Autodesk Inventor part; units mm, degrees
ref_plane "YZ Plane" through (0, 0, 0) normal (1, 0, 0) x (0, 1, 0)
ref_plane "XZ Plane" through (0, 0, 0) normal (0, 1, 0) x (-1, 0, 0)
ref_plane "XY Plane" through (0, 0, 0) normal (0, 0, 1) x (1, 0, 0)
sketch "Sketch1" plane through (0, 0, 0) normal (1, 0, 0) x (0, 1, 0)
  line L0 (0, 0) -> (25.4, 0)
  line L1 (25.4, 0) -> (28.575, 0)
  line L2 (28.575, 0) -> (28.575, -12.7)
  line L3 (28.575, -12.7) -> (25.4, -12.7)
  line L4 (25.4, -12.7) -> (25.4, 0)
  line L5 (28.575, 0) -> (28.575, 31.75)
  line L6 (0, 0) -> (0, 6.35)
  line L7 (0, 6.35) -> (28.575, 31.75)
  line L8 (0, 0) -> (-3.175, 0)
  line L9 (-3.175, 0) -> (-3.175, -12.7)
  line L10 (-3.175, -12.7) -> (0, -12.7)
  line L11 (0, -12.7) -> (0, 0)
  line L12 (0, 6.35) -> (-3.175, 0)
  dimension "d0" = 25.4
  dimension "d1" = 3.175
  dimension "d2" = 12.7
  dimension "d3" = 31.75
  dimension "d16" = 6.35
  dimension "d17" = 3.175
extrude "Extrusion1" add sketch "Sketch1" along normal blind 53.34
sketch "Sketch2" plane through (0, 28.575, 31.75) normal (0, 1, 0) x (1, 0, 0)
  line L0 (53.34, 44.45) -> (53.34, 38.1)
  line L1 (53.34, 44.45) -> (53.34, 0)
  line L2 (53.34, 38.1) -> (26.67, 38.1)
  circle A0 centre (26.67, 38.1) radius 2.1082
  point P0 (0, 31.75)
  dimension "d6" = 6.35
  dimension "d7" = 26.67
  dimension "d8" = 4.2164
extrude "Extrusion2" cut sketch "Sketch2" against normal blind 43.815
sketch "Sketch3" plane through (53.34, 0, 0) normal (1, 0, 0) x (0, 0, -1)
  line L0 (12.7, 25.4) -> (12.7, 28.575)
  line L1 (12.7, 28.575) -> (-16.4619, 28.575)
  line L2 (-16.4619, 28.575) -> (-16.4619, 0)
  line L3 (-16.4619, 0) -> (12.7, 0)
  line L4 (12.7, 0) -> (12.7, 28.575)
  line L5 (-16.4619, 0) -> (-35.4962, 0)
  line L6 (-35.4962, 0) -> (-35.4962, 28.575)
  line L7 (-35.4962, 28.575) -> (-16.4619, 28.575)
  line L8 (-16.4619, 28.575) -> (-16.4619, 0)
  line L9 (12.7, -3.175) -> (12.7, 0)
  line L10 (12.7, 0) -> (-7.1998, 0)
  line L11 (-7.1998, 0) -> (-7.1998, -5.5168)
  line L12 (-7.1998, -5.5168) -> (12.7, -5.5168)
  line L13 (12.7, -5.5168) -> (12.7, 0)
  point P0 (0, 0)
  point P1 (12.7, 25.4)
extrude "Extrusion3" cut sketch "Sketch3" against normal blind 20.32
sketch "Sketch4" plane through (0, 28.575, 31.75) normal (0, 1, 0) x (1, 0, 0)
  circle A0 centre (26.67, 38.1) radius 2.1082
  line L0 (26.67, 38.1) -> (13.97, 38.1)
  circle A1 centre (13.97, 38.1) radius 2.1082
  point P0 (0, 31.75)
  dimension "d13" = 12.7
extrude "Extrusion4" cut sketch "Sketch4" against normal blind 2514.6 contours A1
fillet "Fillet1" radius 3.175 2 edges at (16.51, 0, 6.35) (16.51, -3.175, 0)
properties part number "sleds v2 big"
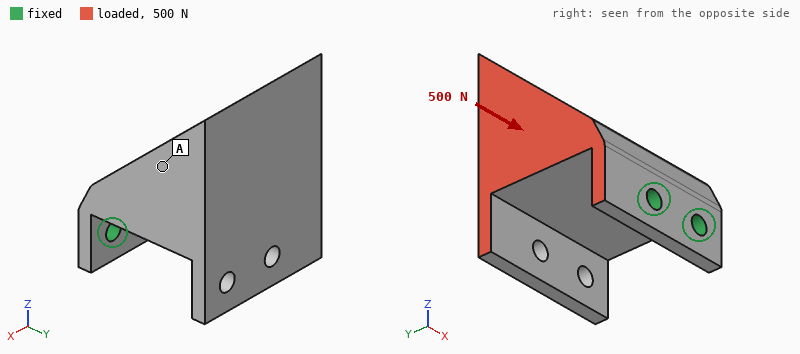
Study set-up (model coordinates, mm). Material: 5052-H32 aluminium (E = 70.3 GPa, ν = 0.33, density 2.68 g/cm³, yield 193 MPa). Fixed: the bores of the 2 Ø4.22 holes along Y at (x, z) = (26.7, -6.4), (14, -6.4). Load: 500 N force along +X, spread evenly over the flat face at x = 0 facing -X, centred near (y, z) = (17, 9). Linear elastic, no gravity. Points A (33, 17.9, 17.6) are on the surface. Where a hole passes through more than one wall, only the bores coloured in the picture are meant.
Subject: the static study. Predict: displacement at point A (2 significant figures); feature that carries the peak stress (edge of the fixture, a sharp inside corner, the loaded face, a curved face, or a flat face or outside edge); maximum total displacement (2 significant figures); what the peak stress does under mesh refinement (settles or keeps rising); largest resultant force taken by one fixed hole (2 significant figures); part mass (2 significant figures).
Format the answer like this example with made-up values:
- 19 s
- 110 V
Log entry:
- 40 µm
- edge of the fixture
- 71 µm
- keeps rising
- 750 N
- 56 g
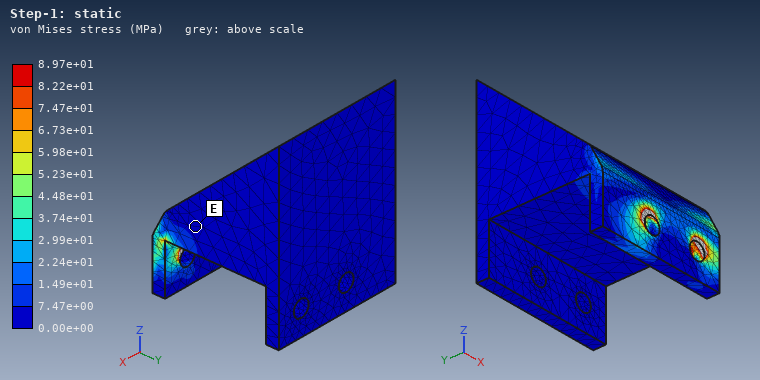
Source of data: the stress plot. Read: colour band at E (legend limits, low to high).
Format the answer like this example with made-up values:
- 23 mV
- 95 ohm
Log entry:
- 0.00e+00 to 7.47e+00 MPa
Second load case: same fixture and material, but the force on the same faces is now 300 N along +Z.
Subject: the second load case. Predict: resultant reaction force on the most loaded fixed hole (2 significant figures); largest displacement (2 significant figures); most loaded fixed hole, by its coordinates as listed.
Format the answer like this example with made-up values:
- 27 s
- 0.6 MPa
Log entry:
- 520 N
- 0.36 mm
- (14, -6.4)
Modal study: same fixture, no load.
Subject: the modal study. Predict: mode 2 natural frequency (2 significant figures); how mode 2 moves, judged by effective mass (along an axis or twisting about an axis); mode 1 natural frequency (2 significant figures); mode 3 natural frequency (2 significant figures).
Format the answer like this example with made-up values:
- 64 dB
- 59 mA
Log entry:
- 2100 Hz
- along X
- 730 Hz
- 5600 Hz
